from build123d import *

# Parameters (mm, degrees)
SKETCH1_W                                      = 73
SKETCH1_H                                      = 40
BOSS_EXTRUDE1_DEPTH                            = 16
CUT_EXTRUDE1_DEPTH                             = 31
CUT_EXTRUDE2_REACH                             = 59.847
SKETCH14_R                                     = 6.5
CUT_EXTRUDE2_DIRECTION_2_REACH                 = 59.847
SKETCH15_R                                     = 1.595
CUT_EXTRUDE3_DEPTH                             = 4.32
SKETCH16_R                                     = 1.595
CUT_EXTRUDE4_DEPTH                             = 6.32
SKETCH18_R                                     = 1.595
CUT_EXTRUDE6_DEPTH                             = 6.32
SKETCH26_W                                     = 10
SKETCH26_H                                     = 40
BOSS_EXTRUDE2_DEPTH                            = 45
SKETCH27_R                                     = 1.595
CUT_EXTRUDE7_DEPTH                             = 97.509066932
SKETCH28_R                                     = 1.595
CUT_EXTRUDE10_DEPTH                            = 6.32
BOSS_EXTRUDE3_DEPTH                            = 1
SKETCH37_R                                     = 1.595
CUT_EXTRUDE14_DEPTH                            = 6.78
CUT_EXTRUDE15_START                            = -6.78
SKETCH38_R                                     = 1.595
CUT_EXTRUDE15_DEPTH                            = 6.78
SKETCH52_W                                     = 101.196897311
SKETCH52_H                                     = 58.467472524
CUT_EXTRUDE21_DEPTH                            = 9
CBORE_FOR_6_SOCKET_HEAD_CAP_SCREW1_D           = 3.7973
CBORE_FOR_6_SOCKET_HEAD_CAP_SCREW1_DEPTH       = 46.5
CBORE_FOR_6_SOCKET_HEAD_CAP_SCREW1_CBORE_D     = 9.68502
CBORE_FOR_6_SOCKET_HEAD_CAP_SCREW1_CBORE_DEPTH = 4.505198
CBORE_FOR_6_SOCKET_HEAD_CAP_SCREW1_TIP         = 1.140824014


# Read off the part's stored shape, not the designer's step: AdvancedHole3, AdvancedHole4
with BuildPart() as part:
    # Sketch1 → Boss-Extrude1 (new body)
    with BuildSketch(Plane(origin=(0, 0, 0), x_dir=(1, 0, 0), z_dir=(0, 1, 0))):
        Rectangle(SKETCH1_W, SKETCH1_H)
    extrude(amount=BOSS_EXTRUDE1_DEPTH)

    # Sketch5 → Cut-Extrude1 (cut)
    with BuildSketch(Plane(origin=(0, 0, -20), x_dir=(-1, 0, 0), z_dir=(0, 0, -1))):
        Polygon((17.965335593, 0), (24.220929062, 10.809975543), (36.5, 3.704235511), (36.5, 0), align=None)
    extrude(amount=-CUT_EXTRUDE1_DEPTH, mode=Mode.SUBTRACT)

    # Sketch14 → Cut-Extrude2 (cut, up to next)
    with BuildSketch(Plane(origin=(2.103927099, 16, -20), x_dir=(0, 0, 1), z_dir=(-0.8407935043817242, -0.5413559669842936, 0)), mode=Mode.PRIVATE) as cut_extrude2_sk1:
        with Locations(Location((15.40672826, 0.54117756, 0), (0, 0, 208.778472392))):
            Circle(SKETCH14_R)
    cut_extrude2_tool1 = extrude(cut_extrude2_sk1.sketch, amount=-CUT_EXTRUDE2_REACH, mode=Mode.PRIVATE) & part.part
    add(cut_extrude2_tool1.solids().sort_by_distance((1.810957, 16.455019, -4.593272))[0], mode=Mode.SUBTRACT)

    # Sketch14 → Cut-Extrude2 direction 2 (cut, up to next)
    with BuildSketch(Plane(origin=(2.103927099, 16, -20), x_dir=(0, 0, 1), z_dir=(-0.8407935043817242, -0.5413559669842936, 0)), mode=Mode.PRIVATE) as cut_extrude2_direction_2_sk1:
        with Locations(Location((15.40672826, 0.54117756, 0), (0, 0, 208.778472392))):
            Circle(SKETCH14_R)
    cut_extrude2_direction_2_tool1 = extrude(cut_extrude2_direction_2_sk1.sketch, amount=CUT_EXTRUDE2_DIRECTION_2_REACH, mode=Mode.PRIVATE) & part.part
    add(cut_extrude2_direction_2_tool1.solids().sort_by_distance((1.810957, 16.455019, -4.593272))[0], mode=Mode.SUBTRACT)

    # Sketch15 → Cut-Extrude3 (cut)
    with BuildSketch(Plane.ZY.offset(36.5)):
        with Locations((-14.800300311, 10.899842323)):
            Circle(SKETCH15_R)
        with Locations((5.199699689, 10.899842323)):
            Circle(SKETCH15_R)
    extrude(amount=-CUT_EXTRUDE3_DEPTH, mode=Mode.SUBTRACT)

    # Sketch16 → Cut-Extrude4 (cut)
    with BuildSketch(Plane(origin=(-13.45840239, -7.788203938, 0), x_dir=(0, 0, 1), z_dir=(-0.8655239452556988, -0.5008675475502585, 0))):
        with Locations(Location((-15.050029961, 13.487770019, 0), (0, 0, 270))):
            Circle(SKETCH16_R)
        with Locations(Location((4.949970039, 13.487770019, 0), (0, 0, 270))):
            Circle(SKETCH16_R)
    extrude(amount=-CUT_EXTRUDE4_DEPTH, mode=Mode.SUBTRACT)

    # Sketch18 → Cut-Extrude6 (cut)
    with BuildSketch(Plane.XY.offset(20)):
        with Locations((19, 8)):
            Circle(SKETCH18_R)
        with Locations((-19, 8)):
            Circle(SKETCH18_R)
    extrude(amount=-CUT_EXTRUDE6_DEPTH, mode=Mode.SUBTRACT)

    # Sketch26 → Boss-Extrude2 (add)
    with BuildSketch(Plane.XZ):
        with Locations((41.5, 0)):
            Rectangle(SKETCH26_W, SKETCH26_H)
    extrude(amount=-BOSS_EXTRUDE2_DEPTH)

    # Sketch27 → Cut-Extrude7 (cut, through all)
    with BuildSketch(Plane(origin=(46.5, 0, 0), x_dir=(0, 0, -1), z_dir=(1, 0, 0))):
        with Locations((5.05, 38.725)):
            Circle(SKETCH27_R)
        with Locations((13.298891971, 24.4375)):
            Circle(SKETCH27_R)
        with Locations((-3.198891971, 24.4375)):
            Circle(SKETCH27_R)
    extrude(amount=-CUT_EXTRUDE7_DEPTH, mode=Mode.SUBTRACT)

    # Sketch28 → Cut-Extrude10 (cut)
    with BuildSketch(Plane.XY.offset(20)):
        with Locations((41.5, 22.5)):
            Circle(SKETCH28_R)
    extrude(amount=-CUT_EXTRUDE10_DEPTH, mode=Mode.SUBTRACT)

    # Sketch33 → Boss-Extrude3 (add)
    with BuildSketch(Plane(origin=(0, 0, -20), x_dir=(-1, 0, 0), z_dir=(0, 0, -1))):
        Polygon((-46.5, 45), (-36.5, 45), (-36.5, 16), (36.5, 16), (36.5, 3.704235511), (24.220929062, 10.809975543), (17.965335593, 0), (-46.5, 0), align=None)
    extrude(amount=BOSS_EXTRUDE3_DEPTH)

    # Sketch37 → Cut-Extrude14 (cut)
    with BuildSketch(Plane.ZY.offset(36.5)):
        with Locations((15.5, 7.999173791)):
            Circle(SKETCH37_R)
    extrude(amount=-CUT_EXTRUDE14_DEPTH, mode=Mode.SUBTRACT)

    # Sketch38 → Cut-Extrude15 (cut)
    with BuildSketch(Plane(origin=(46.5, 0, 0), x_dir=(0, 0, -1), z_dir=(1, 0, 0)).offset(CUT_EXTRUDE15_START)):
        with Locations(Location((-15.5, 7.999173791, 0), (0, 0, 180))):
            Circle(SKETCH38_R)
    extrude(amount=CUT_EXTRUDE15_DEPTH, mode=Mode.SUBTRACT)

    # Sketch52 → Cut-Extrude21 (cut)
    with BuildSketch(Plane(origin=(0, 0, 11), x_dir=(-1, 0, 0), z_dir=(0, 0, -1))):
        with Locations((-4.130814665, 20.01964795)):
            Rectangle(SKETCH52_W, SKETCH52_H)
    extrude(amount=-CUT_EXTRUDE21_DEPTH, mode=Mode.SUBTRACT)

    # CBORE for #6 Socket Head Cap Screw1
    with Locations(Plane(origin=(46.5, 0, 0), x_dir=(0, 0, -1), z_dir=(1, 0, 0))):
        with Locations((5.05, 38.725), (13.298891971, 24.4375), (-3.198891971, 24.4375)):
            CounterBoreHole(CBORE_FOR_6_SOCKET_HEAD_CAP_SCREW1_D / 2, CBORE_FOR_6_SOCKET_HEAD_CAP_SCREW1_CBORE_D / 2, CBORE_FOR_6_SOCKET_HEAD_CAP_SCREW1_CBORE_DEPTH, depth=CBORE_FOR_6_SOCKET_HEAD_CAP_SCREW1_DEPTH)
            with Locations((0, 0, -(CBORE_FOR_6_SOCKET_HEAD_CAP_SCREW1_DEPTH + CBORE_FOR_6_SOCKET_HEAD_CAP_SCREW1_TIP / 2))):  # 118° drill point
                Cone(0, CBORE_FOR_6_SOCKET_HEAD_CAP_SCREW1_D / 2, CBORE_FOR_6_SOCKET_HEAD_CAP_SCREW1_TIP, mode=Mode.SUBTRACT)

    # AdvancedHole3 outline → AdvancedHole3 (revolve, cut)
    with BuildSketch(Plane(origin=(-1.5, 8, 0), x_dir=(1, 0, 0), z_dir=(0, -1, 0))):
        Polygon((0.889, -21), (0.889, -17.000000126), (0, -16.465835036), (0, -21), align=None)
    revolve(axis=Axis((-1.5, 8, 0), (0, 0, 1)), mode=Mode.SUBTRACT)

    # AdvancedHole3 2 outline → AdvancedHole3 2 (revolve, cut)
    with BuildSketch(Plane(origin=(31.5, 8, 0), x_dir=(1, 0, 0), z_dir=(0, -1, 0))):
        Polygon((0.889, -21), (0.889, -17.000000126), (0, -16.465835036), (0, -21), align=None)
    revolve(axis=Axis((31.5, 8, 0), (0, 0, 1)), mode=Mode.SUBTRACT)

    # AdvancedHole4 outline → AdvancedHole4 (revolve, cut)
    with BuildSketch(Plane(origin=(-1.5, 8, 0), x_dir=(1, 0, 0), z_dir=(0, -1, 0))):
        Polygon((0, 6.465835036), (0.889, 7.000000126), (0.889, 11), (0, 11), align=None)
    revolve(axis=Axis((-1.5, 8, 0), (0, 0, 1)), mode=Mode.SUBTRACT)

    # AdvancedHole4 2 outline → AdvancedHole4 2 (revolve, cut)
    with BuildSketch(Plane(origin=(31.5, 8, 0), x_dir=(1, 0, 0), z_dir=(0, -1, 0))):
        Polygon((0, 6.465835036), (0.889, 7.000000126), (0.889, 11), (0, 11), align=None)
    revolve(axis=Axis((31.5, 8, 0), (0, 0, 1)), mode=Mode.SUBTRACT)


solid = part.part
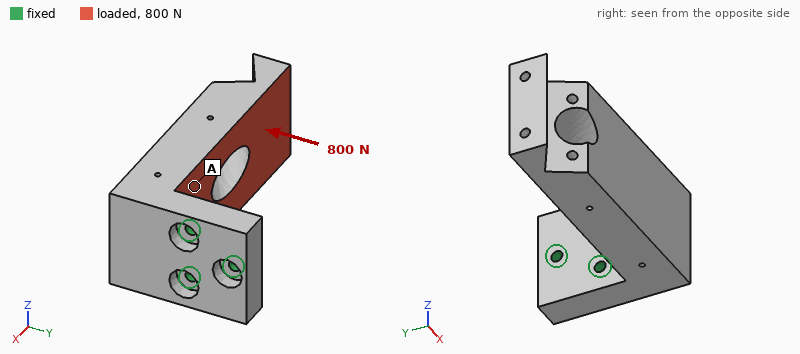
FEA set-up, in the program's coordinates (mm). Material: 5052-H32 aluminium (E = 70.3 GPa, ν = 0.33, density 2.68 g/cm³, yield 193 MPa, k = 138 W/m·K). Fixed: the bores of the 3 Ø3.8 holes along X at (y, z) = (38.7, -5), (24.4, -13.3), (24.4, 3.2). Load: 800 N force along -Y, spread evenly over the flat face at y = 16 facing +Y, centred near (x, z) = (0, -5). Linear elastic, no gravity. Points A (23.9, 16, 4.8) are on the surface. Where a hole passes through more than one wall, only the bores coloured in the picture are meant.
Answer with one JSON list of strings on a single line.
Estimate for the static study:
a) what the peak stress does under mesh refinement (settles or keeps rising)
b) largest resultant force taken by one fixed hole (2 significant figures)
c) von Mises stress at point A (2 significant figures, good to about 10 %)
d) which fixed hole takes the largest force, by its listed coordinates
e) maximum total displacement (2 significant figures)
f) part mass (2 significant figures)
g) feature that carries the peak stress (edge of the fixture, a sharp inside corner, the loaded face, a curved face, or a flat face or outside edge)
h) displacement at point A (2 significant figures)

["keeps rising", "1.3 kN", "14 MPa", "(38.7, -5)", "0.36 mm", "120 g", "edge of the fixture", "0.067 mm"]
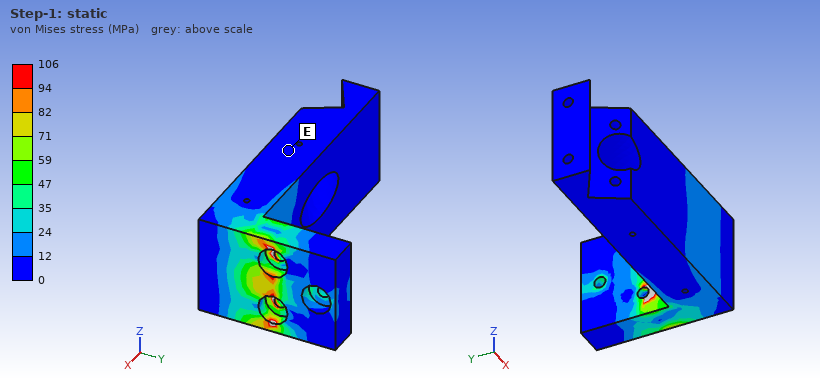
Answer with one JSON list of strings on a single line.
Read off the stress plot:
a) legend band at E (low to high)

["0 to 12 MPa"]
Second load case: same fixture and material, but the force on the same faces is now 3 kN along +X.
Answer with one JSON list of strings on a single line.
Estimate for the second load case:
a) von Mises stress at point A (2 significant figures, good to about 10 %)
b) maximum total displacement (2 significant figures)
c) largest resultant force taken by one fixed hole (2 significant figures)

["19 MPa", "56 µm", "1.9 kN"]
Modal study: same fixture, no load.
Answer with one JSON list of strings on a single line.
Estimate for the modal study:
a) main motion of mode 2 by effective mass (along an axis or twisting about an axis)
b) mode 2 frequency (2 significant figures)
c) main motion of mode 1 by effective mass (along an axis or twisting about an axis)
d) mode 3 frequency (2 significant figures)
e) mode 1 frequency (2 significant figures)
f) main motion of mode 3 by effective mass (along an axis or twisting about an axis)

["along Z", "1900 Hz", "along Y", "6000 Hz", "1100 Hz", "along X"]
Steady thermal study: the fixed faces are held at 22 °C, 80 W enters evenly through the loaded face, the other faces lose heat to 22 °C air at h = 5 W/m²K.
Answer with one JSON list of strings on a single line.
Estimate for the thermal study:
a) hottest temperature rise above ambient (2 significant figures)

["83 K"]
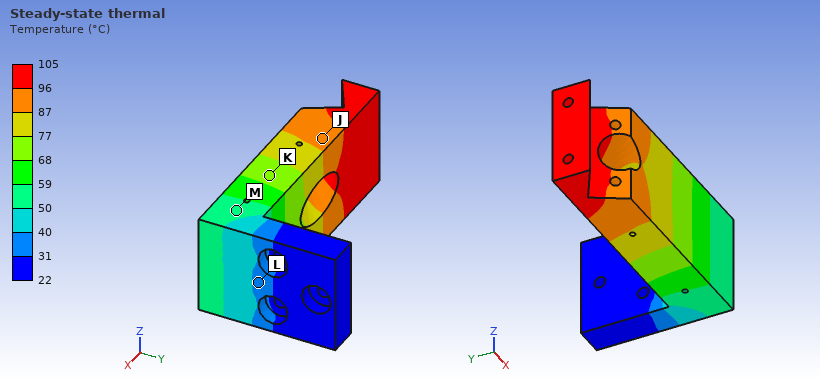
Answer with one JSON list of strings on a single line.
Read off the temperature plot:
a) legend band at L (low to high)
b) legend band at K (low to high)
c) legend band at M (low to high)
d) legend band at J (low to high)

["31 to 40 °C", "68 to 77 °C", "50 to 59 °C", "87 to 96 °C"]
